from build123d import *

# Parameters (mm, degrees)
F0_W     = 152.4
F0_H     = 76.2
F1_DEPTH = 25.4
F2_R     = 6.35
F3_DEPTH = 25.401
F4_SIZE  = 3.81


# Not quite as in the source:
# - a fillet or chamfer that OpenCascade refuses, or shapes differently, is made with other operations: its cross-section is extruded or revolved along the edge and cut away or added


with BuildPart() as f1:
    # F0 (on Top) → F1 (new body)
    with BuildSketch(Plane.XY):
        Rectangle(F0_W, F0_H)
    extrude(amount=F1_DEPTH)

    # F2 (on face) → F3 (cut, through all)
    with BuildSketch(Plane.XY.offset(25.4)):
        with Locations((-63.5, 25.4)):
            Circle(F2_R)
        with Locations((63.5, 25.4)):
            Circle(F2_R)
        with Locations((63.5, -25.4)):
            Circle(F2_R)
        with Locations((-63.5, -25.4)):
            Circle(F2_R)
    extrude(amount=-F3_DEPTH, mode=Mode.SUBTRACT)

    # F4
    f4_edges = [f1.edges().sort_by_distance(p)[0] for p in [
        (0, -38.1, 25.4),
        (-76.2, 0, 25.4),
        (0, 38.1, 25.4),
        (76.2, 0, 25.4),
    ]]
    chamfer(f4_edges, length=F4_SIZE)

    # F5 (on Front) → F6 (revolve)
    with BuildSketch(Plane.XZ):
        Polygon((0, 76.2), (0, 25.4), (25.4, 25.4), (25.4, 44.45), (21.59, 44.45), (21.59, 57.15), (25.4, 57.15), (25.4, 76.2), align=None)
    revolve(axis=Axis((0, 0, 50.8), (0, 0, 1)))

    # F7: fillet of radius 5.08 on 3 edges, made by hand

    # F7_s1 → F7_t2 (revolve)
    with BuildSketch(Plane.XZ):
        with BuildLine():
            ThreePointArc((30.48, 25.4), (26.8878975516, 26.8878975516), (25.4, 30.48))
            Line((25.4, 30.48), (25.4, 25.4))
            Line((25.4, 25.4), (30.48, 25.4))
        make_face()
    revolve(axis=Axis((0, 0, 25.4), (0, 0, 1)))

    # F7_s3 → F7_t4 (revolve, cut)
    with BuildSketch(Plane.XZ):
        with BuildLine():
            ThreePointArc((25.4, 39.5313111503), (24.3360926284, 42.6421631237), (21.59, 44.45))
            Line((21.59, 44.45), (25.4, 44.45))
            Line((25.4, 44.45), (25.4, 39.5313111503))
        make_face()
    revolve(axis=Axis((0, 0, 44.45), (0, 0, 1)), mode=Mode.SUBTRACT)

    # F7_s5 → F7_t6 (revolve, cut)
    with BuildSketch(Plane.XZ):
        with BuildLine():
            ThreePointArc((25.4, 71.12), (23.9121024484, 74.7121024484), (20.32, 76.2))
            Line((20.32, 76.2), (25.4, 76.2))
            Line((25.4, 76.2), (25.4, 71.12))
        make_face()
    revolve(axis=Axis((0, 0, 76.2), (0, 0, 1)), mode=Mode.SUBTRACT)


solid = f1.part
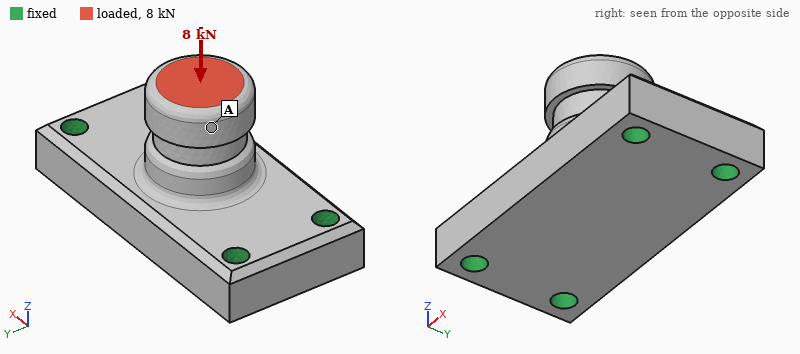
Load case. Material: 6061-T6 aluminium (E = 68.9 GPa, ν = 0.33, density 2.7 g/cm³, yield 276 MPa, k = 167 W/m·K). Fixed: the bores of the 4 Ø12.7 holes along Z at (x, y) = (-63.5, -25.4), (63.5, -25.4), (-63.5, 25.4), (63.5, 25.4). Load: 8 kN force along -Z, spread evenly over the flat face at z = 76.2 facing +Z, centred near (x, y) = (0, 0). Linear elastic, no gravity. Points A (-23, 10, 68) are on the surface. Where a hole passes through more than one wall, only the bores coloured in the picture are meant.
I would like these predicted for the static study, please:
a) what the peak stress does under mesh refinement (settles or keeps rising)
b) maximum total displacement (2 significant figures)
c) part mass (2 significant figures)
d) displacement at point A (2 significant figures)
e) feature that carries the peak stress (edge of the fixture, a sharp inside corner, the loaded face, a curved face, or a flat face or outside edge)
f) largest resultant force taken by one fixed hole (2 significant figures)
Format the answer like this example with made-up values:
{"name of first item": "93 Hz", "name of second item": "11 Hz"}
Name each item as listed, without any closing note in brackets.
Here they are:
{"what the peak stress does under mesh refinement": "keeps rising", "maximum total displacement": "14 µm", "part mass": "1.0 kg", "displacement at point A": "13 µm", "feature that carries the peak stress": "edge of the fixture", "largest resultant force taken by one fixed hole": "2.1 kN"}
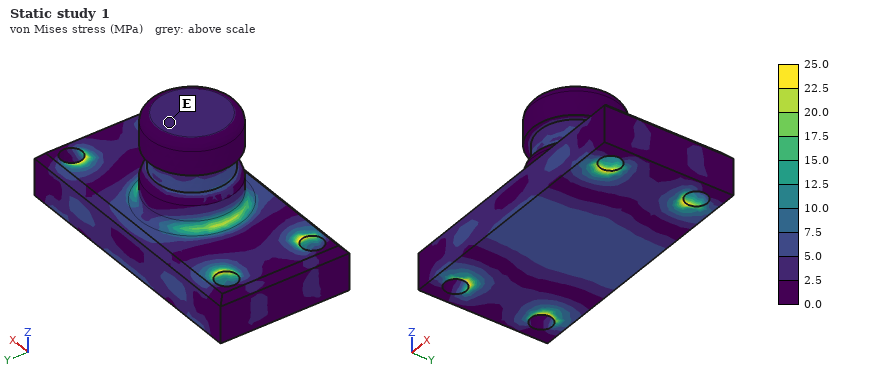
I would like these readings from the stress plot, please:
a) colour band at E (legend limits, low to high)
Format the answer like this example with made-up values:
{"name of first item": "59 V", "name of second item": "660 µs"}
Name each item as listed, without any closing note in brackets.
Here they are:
{"colour band at E": "2.5 to 5.0 MPa"}
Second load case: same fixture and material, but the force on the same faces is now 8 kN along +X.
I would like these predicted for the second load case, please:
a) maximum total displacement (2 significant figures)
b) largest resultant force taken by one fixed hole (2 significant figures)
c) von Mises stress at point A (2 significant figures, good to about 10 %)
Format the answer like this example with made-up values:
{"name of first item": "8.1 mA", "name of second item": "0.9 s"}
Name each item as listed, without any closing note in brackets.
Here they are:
{"maximum total displacement": "56 µm", "largest resultant force taken by one fixed hole": "3.4 kN", "von Mises stress at point A": "5.1 MPa"}
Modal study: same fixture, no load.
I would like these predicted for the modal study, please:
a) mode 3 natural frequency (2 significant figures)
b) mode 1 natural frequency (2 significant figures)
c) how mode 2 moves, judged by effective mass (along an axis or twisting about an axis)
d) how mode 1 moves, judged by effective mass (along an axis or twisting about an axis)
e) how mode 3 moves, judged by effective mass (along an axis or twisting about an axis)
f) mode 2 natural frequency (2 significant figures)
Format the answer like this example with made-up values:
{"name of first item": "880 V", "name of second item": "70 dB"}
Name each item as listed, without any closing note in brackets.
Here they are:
{"mode 3 natural frequency": "6300 Hz", "mode 1 natural frequency": "4300 Hz", "how mode 2 moves, judged by effective mass": "along Z", "how mode 1 moves, judged by effective mass": "along Y", "how mode 3 moves, judged by effective mass": "along X", "mode 2 natural frequency": "5600 Hz"}
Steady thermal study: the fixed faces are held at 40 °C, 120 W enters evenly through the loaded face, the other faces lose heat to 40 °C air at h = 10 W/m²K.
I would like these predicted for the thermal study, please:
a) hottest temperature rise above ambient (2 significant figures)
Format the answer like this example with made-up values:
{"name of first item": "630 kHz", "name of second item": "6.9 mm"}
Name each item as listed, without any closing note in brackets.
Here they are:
{"hottest temperature rise above ambient": "33 K"}
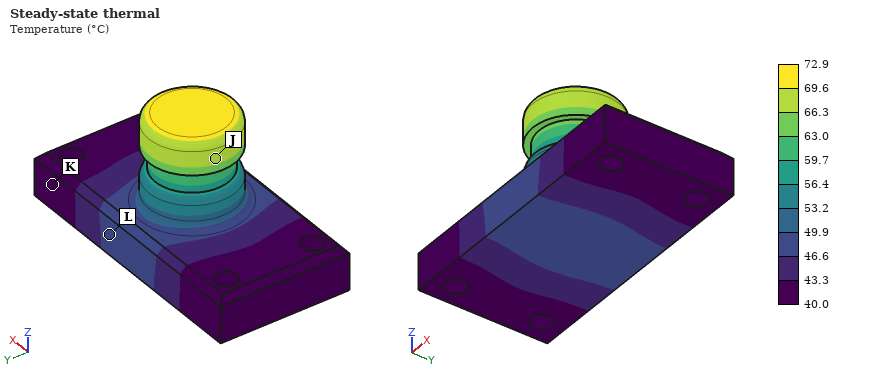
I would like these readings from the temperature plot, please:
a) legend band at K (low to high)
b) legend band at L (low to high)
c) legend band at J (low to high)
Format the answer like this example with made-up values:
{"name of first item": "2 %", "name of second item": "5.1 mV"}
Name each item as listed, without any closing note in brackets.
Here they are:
{"legend band at K": "40.0 to 43.3 °C", "legend band at L": "46.6 to 49.9 °C", "legend band at J": "66.3 to 69.6 °C"}
